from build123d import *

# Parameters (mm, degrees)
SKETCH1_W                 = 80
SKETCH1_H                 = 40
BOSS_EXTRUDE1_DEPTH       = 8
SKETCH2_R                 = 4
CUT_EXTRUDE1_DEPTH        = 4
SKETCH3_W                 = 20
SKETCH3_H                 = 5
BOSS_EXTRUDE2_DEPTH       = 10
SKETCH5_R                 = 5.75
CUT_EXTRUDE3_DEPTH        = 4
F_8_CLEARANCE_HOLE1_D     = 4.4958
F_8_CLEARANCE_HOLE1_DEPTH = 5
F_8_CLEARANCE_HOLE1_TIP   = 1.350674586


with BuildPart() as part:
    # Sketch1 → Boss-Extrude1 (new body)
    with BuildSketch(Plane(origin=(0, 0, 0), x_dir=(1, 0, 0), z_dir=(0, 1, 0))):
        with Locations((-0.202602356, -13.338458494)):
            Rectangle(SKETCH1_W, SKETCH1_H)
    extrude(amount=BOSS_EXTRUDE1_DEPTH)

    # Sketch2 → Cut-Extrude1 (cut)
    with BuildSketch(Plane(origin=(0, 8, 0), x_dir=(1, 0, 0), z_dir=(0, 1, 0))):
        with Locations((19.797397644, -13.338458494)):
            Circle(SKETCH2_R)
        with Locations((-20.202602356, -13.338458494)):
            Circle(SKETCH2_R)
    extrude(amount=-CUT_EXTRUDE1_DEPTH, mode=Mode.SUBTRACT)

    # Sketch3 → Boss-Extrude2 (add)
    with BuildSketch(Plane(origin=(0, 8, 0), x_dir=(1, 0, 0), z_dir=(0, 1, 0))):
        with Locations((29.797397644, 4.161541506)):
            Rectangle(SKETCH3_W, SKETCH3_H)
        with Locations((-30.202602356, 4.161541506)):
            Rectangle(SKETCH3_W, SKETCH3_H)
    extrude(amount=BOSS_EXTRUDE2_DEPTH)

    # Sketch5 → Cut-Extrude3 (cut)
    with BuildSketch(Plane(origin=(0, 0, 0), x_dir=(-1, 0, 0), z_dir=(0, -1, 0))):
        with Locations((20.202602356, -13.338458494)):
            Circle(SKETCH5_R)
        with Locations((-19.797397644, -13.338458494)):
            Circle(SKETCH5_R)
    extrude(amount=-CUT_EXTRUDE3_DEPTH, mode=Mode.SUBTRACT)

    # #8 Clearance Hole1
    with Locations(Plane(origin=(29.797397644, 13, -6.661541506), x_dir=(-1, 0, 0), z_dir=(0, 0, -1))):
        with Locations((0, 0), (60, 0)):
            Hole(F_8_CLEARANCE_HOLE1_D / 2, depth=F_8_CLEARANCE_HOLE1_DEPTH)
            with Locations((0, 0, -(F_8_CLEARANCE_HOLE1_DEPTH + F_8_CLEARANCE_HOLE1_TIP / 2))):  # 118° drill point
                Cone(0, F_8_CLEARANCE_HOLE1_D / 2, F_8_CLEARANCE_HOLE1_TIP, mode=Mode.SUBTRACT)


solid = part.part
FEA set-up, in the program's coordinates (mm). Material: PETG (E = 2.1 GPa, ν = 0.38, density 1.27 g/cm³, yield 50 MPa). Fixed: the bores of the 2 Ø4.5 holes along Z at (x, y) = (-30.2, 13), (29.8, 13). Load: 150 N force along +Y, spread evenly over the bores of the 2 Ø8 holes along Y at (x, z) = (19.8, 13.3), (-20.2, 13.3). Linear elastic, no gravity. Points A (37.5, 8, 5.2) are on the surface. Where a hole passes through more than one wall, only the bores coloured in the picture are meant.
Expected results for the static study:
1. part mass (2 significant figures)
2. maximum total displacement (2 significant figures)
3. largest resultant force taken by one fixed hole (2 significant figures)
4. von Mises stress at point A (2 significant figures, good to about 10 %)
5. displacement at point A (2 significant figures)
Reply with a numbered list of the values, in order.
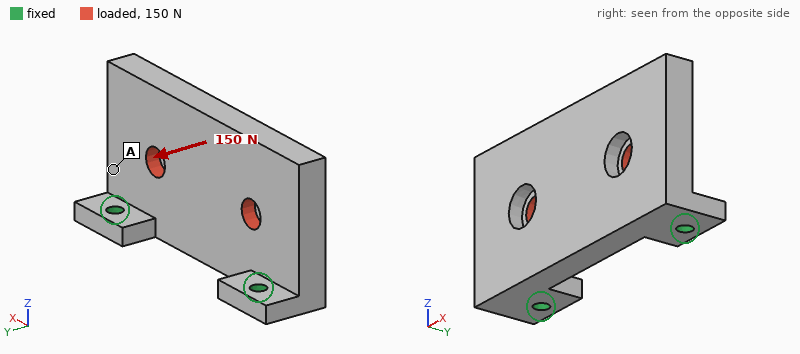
1. 33 g
2. 1.0 mm
3. 83 N
4. 2.3 MPa
5. 0.19 mm
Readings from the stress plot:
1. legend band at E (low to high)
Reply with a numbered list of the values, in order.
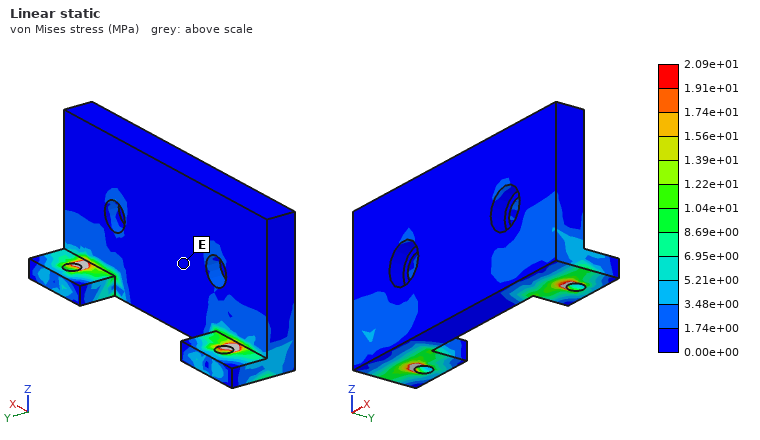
1. 0.00e+00 to 1.74e+00 MPa
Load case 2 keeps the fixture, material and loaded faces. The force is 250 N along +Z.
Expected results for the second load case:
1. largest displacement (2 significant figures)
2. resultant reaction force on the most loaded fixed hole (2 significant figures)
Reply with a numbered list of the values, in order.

1. 0.25 mm
2. 130 N
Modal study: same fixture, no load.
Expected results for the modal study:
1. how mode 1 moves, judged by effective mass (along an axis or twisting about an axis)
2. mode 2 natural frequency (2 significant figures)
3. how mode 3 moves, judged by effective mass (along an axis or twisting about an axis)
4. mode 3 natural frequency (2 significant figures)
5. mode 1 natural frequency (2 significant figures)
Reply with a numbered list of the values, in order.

1. along Y
2. 1100 Hz
3. along X
4. 1900 Hz
5. 420 Hz
